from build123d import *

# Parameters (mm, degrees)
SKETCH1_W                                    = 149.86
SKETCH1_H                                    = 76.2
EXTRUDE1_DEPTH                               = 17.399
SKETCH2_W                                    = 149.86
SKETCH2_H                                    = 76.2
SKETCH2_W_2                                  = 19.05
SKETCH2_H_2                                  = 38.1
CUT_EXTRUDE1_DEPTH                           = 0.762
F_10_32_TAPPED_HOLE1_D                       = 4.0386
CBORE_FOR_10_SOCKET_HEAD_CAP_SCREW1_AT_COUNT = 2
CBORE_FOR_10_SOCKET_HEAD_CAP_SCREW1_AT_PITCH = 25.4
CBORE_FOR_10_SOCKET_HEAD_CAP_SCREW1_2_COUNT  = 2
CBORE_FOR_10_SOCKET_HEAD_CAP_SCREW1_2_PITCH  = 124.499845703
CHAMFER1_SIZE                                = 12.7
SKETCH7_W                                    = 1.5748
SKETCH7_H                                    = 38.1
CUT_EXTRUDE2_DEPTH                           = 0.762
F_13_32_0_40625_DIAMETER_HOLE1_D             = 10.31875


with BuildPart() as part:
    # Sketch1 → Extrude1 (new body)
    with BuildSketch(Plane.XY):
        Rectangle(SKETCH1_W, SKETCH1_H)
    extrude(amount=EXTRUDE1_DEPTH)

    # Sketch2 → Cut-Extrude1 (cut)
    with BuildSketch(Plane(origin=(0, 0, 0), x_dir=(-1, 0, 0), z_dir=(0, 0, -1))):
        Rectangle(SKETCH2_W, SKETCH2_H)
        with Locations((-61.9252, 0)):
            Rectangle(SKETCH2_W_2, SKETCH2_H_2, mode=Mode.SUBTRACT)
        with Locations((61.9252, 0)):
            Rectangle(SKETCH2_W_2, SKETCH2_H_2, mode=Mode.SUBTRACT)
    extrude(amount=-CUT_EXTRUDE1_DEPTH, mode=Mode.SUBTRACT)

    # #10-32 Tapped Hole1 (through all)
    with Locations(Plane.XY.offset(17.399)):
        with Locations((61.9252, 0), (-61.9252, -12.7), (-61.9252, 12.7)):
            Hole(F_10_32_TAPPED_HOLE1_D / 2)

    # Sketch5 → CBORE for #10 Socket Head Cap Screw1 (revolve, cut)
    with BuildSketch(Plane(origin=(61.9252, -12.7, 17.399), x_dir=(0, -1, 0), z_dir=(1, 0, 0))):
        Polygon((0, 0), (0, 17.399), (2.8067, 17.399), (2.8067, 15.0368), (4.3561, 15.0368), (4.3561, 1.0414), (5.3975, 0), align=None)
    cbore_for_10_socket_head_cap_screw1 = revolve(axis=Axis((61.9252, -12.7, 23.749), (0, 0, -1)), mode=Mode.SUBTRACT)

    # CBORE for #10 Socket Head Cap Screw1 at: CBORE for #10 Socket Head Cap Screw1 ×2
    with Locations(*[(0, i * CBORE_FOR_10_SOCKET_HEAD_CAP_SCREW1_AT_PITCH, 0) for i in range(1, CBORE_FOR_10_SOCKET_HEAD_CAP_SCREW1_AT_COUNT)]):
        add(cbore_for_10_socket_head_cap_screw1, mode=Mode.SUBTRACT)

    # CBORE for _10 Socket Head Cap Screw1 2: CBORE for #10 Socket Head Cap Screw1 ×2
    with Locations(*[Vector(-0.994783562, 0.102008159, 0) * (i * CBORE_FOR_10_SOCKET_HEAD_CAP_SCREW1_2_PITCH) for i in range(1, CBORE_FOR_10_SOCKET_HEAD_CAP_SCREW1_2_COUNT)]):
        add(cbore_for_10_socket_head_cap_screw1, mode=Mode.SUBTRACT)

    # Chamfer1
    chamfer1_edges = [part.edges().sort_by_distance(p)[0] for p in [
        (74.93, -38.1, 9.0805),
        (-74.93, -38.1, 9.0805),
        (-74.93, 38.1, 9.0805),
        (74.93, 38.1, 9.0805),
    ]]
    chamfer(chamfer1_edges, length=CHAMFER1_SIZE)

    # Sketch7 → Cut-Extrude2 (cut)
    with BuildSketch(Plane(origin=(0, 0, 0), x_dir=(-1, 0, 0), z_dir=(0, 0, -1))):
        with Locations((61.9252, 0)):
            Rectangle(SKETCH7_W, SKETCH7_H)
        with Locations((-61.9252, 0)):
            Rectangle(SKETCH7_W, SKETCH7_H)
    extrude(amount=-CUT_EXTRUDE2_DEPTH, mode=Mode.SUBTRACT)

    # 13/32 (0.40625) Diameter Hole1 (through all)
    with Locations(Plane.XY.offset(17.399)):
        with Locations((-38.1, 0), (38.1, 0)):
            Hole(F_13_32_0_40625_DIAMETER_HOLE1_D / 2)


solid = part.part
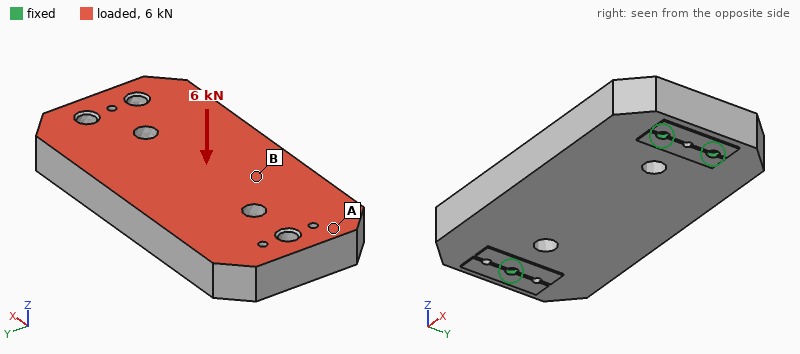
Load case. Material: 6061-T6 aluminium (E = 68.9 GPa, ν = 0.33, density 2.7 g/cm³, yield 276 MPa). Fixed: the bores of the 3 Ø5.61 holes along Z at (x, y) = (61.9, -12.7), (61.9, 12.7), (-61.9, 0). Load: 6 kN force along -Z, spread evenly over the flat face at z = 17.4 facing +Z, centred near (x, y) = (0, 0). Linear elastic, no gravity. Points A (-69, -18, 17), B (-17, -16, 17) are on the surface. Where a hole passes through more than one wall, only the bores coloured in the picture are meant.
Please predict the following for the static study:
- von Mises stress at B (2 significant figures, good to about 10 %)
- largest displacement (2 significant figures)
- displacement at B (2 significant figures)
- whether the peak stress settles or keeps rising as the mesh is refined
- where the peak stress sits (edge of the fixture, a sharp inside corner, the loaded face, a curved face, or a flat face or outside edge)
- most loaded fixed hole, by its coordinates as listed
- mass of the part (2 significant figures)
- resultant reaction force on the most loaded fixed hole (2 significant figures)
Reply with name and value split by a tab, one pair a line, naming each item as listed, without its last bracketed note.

von Mises stress at B	16 MPa
largest displacement	52 µm
displacement at B	44 µm
whether the peak stress settles or keeps rising as the mesh is refined	keeps rising
where the peak stress sits	edge of the fixture
most loaded fixed hole, by its coordinates as listed	(-61.9, 0)
mass of the part	480 g
resultant reaction force on the most loaded fixed hole	4.3 kN
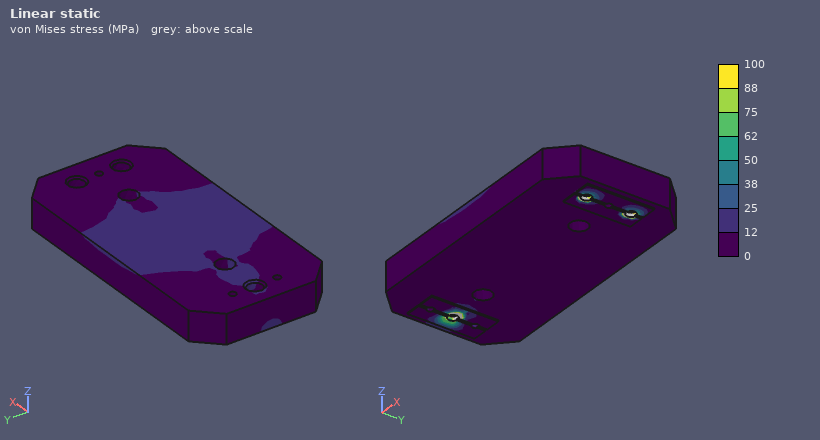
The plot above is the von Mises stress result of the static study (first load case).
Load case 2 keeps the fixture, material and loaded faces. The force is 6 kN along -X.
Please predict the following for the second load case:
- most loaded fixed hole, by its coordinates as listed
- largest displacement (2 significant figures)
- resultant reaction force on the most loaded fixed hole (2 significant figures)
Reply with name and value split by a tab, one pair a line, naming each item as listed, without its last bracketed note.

most loaded fixed hole, by its coordinates as listed	(-61.9, 0)
largest displacement	12 µm
resultant reaction force on the most loaded fixed hole	2.6 kN
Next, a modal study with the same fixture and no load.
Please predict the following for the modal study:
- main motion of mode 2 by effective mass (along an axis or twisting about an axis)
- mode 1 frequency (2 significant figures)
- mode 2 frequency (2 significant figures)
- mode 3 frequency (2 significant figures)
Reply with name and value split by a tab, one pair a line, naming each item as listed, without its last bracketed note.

main motion of mode 2 by effective mass	along Z
mode 1 frequency	2000 Hz
mode 2 frequency	2800 Hz
mode 3 frequency	5700 Hz
